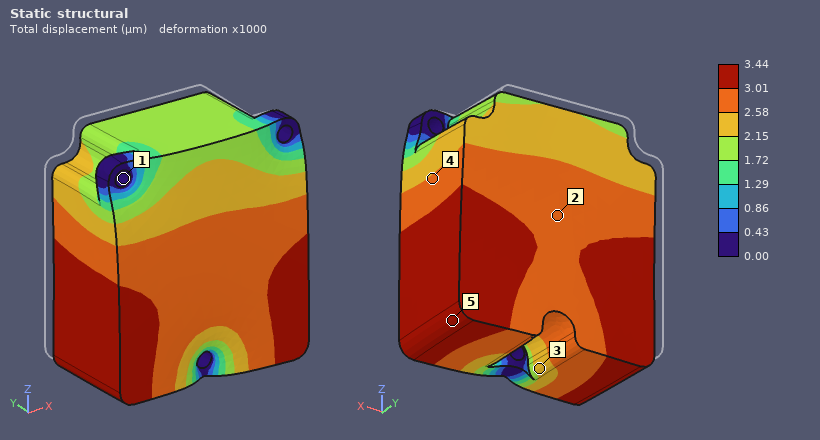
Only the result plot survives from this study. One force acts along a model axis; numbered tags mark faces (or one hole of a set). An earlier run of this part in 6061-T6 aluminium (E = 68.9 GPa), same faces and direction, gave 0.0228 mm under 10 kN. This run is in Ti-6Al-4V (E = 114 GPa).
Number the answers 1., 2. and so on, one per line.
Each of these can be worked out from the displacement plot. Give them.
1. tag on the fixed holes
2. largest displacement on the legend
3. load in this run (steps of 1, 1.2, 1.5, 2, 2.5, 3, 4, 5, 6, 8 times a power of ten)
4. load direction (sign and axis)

1. 1
2. 3.44 µm
3. 2.5 kN
4. -Y
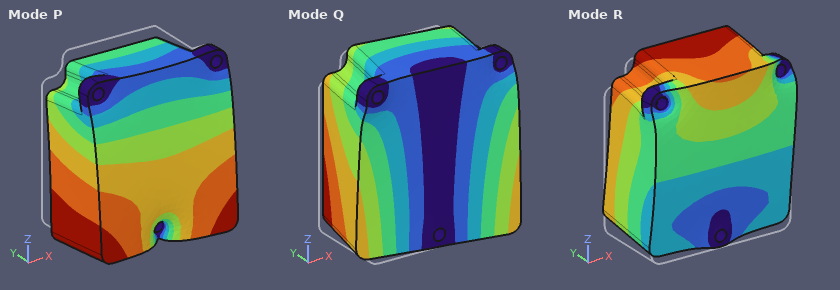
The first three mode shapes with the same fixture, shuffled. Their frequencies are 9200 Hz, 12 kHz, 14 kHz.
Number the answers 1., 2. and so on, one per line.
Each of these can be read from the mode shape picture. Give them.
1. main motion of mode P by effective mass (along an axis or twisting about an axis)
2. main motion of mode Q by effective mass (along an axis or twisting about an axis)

1. along Y
2. along X
